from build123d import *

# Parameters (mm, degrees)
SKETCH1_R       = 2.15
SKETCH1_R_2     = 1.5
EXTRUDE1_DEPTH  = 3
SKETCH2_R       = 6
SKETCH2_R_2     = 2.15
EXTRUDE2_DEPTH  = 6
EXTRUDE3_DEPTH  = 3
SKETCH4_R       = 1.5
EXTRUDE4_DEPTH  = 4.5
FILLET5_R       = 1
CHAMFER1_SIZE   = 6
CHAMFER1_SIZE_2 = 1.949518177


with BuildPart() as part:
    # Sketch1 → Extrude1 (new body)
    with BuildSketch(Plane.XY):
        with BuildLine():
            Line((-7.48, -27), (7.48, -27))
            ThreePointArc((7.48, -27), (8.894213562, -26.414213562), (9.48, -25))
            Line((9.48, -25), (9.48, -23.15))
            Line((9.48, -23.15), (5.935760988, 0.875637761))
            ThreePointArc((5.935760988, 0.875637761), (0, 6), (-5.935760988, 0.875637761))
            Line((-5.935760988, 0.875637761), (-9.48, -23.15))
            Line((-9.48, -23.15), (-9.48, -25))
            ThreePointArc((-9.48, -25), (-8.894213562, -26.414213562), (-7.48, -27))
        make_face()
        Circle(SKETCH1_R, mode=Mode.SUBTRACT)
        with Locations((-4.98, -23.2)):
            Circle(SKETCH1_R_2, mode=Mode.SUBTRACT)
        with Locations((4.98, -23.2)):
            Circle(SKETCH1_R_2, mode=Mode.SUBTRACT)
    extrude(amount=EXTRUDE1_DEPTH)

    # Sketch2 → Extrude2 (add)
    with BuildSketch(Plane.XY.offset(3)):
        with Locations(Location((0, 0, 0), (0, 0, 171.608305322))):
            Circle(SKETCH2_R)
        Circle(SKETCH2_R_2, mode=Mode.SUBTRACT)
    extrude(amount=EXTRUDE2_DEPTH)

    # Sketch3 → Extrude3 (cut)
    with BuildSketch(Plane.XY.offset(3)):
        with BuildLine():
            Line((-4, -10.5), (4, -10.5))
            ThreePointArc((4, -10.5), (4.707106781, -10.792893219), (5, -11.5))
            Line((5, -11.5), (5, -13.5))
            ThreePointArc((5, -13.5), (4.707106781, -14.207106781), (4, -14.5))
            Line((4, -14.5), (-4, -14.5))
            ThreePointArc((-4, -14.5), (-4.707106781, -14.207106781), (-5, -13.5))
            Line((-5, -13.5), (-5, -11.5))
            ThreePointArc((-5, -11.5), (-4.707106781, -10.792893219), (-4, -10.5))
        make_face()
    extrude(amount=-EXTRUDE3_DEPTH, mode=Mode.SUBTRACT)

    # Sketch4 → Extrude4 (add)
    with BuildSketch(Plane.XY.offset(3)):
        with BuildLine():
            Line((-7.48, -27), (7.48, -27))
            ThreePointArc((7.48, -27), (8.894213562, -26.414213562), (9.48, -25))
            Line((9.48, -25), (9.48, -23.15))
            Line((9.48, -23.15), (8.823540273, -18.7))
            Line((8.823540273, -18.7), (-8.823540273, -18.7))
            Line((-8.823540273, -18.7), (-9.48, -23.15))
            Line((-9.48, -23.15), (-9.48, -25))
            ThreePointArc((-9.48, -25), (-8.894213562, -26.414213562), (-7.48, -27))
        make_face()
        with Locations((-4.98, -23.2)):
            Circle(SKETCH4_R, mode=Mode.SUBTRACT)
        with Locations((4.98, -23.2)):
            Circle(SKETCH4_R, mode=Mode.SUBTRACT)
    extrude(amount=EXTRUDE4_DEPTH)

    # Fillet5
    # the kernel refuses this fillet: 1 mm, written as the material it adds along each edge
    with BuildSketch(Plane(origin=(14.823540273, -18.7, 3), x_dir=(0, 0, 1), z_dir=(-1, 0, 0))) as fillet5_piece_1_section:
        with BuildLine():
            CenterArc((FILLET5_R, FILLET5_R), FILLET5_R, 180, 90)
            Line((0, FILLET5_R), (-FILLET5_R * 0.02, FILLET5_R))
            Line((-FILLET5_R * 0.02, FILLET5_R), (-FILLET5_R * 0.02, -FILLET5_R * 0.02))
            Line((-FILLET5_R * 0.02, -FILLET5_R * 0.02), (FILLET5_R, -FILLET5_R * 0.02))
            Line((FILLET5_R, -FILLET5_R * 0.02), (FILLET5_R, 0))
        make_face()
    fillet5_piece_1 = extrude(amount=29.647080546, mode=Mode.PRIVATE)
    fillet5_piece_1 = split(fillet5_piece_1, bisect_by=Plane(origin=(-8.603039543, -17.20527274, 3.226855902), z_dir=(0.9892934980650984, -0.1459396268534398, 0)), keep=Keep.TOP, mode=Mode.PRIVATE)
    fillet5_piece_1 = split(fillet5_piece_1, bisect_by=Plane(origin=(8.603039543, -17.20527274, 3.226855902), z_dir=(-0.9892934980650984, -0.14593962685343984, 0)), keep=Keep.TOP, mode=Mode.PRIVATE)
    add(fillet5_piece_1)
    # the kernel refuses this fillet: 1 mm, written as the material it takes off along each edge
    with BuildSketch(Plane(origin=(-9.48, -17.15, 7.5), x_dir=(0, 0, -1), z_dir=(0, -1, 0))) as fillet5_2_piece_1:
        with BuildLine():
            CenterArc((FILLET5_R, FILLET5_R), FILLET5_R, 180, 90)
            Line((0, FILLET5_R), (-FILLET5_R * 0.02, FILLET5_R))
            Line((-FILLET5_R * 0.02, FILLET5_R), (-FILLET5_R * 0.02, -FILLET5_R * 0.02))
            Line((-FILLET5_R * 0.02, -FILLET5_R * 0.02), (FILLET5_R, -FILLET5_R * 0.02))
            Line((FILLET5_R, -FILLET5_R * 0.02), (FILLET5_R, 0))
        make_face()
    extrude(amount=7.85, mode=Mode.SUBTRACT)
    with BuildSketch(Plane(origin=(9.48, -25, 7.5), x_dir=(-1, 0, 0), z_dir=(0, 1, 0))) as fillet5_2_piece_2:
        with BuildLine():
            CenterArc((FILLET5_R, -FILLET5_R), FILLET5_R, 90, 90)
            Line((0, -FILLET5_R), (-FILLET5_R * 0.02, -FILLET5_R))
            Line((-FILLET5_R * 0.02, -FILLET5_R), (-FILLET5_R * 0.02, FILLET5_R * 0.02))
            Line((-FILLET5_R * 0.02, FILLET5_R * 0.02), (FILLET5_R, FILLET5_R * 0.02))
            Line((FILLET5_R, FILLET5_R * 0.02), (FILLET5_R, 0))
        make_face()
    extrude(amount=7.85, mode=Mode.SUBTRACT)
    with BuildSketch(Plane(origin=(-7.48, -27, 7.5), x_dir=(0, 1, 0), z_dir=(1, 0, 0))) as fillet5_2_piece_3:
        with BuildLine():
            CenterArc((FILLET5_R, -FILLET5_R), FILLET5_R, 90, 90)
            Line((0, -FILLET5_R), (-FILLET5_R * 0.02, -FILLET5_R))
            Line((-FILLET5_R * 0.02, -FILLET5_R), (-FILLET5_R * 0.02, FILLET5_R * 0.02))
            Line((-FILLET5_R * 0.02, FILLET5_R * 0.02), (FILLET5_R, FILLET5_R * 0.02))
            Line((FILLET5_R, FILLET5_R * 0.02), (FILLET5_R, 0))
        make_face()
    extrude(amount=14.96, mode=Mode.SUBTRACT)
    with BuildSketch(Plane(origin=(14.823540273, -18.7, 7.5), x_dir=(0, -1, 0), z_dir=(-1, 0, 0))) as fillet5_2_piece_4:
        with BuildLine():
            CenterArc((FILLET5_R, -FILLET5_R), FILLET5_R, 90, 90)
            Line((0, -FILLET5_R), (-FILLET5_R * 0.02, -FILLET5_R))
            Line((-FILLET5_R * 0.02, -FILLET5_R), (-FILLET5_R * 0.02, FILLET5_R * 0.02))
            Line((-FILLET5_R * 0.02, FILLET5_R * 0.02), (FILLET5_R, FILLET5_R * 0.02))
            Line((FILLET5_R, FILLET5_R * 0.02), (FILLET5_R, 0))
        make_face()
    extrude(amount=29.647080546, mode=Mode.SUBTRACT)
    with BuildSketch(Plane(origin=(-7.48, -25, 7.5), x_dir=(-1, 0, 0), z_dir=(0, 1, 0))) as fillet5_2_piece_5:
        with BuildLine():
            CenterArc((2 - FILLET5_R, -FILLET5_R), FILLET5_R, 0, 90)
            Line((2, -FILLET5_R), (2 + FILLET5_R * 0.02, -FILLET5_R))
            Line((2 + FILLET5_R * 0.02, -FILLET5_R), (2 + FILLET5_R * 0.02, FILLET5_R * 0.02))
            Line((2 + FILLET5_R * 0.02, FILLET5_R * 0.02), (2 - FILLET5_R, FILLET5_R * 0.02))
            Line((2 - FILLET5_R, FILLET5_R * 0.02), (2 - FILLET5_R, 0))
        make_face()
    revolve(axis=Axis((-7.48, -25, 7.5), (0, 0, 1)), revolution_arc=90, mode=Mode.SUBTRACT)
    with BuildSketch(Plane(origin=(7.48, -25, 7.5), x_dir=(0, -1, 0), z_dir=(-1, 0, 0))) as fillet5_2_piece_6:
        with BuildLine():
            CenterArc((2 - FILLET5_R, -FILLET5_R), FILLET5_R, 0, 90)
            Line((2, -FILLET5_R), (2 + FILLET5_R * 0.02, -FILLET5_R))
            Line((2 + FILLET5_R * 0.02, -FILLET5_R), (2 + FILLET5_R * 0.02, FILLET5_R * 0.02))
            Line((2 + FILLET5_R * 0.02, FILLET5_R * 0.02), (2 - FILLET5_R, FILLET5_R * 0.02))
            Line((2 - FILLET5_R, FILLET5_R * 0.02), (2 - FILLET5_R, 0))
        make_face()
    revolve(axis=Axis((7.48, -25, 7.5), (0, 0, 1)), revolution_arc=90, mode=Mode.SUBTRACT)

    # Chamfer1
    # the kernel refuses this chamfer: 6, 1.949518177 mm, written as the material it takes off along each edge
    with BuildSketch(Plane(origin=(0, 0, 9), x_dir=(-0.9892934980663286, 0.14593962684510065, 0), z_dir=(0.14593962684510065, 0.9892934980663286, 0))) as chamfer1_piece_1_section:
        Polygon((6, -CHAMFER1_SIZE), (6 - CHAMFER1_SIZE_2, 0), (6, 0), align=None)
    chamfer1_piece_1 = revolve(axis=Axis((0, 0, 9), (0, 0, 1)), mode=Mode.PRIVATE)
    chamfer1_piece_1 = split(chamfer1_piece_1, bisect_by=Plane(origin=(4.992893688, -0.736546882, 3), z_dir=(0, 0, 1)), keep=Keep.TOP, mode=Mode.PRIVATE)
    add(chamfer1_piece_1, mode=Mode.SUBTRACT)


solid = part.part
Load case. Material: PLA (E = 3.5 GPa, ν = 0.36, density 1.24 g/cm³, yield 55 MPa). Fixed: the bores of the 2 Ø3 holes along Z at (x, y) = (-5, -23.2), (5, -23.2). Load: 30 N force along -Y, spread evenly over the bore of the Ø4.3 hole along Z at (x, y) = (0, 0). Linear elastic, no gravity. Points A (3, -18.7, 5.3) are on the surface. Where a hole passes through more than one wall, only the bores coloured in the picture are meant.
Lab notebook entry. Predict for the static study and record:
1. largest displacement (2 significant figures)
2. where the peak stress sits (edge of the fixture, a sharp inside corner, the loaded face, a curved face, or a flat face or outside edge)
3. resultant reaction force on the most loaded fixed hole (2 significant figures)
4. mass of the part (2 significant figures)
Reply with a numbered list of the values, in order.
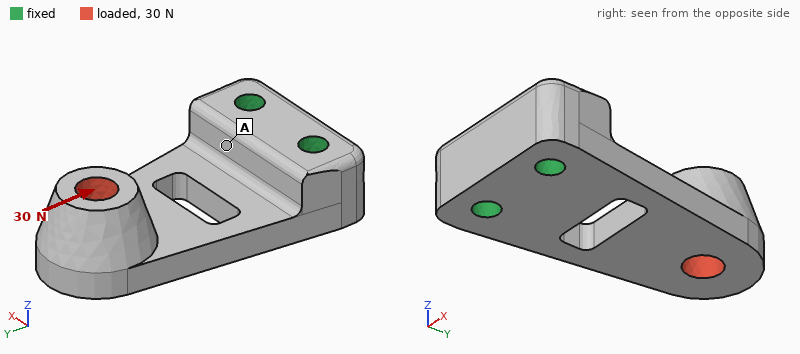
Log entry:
1. 0.38 mm
2. a curved face
3. 15 N
4. 2.8 g
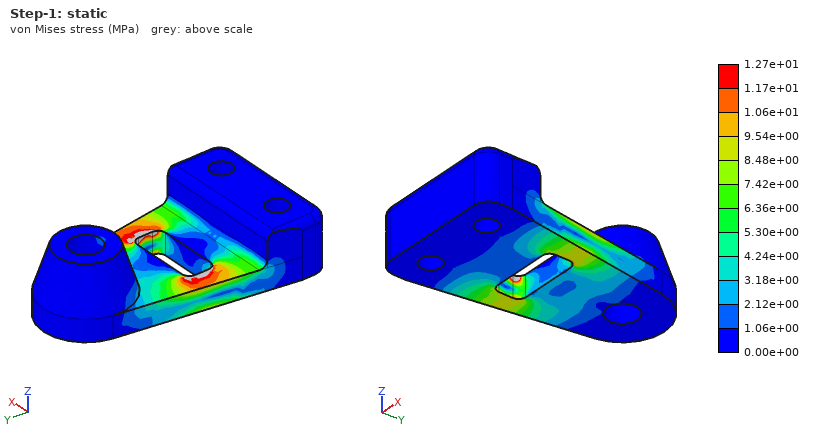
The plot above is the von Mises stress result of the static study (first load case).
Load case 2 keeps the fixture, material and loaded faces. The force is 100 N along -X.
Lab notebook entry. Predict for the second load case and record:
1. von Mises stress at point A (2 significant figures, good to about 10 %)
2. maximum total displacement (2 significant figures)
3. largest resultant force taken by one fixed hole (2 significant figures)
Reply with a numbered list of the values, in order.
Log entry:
1. 3.0 MPa
2. 0.44 mm
3. 190 N
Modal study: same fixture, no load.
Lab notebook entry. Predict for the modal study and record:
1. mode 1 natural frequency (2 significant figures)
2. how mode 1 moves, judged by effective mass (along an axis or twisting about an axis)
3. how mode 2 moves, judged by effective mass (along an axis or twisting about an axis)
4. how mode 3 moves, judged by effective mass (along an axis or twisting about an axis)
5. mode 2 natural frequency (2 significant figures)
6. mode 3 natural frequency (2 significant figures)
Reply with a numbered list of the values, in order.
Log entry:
1. 810 Hz
2. along Z
3. along X
4. along X
5. 2900 Hz
6. 4600 Hz
